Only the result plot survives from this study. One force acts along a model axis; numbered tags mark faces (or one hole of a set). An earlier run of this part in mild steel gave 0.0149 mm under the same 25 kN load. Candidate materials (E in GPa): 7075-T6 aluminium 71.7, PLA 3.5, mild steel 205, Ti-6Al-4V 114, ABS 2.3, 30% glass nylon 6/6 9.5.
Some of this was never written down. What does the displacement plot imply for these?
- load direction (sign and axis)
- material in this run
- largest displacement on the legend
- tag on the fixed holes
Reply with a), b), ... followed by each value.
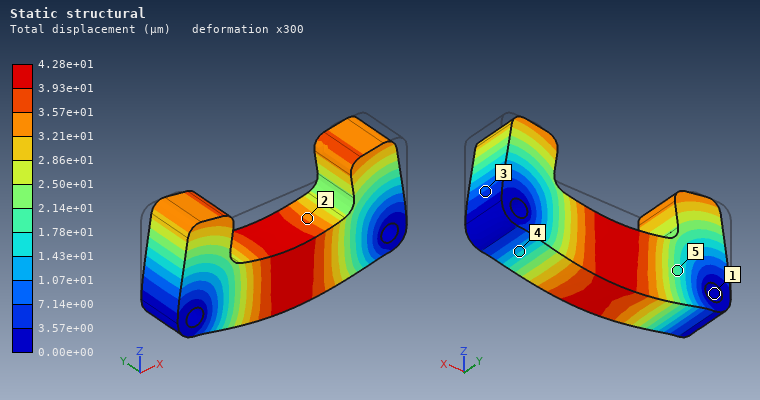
a) -Z
b) 7075-T6 aluminium
c) 4.28e+01 µm
d) 1
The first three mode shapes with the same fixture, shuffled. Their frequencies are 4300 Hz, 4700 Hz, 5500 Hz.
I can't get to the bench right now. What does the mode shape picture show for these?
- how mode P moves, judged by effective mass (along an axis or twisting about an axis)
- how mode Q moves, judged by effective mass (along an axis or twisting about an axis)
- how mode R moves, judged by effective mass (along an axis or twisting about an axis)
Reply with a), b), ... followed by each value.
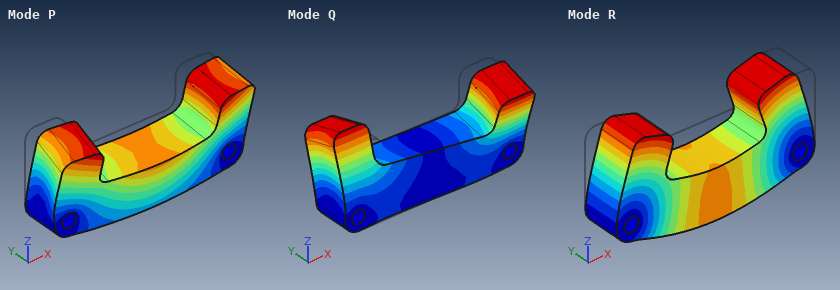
a) along Y
b) twisting about Z
c) along Z
